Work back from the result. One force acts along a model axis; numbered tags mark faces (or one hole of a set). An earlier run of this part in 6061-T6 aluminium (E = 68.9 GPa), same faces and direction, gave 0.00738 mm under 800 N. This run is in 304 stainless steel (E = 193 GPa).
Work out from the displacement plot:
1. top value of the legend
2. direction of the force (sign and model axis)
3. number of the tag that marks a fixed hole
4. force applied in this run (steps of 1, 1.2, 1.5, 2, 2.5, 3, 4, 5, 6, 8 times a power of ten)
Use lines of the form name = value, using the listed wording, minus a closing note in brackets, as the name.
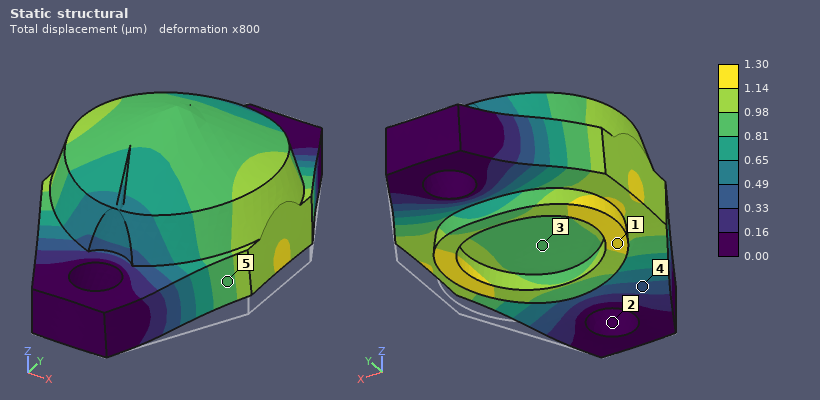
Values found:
top value of the legend = 1.30 µm
direction of the force = +Z
number of the tag that marks a fixed hole = 2
force applied in this run = 400 N
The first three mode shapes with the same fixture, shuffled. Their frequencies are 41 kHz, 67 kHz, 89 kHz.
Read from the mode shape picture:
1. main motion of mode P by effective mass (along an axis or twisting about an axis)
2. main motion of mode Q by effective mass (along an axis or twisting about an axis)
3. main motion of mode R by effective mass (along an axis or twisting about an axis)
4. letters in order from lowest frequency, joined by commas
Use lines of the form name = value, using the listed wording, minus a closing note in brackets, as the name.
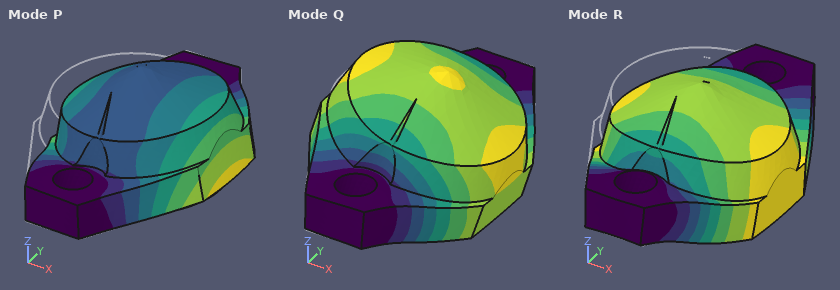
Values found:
main motion of mode P by effective mass = along X
main motion of mode Q by effective mass = along X
main motion of mode R by effective mass = along Z
letters in order from lowest frequency, joined by commas = Q, R, P
